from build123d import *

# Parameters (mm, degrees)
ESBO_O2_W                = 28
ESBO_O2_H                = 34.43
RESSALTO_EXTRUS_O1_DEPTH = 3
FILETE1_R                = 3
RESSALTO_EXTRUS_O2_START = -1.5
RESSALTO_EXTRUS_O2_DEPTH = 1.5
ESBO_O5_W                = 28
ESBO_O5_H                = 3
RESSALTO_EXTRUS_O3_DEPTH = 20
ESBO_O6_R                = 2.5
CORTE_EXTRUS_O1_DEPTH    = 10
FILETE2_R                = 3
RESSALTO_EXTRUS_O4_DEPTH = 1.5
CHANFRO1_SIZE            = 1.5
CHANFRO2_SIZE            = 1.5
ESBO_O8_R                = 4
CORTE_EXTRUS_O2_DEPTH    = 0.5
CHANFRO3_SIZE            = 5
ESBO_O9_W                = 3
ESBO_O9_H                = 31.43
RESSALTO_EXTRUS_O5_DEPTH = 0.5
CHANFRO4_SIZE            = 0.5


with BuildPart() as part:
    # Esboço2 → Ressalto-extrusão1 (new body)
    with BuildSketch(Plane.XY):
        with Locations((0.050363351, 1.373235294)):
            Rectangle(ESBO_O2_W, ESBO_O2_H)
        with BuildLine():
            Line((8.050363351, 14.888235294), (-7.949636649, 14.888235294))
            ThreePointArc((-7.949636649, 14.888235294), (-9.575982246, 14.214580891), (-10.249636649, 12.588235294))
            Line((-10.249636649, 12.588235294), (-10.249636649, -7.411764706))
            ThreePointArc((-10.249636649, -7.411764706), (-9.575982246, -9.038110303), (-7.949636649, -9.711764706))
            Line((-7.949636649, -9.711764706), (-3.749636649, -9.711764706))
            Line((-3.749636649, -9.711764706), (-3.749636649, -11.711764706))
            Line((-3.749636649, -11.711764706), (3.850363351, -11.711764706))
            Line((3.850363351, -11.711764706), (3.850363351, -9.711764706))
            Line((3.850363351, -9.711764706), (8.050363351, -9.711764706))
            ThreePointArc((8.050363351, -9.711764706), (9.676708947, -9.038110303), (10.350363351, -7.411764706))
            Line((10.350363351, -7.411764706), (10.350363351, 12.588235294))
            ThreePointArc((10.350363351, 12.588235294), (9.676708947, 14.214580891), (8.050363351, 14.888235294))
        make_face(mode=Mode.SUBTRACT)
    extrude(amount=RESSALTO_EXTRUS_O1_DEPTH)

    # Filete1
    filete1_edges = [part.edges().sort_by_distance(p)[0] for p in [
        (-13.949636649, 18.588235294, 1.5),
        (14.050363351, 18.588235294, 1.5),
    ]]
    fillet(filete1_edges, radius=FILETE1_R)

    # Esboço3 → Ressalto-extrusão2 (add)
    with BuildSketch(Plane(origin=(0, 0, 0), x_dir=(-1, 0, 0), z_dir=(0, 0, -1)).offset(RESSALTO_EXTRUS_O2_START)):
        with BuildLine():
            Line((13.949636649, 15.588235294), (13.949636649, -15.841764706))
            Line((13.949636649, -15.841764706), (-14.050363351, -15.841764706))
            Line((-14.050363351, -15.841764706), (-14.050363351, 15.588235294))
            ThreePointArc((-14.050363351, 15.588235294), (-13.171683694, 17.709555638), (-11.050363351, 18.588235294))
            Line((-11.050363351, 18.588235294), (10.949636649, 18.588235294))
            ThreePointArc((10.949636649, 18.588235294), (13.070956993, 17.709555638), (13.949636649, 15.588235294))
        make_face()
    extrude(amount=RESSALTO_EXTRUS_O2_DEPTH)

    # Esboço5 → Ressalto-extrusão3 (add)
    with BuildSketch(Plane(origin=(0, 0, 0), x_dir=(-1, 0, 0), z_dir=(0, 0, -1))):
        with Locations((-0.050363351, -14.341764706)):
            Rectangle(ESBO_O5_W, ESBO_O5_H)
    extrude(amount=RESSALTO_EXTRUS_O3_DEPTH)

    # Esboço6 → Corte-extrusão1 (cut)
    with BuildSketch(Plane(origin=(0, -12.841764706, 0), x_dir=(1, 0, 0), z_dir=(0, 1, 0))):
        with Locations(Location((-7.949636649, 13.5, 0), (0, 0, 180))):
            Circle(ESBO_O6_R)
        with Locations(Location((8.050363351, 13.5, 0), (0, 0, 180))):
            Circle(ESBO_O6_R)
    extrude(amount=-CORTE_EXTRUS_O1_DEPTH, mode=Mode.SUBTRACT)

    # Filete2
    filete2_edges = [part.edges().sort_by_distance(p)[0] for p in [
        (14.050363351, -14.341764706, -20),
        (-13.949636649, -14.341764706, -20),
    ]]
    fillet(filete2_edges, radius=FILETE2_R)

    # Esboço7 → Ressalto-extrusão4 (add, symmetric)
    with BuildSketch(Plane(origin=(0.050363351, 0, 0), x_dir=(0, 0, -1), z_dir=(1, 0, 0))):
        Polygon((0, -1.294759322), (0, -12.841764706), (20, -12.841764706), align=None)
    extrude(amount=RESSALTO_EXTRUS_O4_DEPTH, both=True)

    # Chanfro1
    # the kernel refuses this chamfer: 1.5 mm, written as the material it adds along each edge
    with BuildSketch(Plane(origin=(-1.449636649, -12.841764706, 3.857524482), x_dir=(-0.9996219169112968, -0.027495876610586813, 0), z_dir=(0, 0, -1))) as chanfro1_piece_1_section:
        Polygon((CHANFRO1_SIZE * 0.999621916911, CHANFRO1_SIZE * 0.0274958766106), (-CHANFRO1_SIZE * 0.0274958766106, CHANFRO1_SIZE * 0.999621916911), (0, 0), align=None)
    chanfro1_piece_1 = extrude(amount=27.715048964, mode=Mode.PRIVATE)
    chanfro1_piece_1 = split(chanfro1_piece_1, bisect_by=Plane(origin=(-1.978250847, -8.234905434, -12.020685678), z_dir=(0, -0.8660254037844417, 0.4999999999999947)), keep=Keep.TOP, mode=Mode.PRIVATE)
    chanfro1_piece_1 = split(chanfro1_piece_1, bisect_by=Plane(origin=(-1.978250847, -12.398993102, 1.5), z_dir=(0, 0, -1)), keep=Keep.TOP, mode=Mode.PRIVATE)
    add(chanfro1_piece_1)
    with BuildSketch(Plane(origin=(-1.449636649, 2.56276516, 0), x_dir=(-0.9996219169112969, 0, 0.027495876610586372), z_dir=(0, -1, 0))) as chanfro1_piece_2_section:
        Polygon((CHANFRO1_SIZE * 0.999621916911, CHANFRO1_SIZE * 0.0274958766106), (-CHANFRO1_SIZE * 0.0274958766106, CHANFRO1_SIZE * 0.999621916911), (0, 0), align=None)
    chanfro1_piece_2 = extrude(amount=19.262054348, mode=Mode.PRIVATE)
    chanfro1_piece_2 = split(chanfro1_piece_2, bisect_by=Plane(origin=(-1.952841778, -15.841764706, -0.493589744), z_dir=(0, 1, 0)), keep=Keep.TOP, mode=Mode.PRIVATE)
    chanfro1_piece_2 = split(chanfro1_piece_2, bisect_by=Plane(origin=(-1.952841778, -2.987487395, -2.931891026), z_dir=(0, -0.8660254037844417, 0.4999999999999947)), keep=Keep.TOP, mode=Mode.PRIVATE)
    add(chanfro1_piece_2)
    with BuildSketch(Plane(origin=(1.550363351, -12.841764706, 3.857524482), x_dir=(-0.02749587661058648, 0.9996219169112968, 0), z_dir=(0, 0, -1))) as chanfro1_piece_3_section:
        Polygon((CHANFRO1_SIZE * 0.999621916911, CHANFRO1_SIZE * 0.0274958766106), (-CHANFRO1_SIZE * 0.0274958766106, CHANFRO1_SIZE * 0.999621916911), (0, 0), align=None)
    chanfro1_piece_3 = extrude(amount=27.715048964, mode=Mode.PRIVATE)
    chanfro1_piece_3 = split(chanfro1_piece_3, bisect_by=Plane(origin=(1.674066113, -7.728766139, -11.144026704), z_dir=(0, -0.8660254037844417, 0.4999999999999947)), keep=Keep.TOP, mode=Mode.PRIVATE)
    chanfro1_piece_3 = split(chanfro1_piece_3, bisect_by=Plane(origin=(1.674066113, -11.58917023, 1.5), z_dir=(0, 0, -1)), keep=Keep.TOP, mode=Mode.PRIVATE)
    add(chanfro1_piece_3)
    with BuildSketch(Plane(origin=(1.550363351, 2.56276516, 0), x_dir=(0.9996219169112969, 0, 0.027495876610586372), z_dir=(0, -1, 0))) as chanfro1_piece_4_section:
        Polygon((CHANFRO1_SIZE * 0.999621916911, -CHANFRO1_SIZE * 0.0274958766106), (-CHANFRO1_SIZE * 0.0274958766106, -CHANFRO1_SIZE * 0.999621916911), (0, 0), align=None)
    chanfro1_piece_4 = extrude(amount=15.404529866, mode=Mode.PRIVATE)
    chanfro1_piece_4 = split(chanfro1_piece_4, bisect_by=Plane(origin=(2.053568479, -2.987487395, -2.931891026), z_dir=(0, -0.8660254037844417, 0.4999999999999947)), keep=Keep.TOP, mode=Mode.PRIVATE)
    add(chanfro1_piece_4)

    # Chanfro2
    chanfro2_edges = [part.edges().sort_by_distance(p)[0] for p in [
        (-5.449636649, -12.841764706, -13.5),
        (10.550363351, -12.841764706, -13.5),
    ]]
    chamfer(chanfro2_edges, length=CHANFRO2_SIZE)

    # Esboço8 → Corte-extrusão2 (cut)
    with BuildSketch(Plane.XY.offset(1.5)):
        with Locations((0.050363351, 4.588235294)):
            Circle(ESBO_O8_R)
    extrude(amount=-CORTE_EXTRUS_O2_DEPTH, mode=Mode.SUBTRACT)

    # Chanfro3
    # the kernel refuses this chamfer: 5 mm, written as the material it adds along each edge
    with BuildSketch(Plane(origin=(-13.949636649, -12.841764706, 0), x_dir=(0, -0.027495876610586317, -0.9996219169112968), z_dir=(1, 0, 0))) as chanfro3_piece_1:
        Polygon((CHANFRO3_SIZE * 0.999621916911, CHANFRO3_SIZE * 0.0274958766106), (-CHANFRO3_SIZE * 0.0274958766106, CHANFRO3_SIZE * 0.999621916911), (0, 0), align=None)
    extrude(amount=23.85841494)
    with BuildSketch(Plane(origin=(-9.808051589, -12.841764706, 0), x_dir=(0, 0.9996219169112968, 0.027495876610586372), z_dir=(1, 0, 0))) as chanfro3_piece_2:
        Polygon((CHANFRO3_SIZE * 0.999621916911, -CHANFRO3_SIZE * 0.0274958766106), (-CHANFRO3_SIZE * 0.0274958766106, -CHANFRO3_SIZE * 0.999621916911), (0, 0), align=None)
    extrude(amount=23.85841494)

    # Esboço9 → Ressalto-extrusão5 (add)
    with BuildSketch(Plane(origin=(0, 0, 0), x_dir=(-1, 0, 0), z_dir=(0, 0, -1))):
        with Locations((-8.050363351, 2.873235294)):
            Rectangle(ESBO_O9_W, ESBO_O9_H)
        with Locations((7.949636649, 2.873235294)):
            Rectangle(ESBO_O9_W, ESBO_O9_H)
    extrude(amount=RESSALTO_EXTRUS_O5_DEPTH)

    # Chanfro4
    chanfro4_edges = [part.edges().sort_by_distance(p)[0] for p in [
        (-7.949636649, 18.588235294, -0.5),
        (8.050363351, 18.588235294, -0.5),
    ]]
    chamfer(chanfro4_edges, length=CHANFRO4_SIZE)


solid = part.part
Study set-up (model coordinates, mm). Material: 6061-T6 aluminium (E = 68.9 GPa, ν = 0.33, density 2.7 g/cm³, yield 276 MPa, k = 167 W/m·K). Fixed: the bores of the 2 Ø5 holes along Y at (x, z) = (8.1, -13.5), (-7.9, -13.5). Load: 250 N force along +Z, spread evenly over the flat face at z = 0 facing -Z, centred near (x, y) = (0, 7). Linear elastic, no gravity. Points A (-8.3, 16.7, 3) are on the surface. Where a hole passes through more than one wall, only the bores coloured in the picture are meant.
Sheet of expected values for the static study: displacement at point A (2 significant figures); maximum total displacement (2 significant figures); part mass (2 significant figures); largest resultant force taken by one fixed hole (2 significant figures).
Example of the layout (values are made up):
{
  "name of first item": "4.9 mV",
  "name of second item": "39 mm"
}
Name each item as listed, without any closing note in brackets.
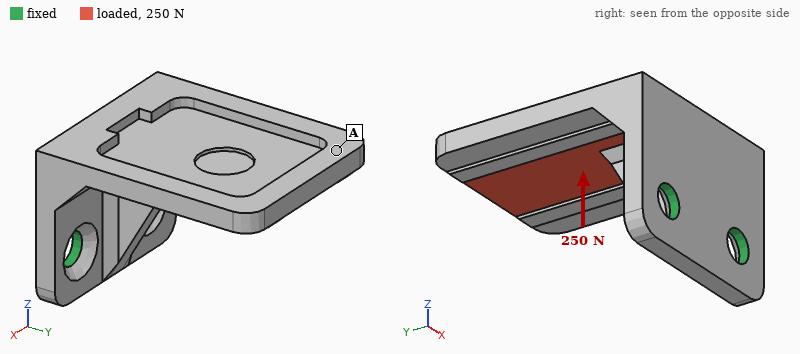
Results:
{
  "displacement at point A": "0.41 mm",
  "maximum total displacement": "0.45 mm",
  "part mass": "12 g",
  "largest resultant force taken by one fixed hole": "130 N"
}
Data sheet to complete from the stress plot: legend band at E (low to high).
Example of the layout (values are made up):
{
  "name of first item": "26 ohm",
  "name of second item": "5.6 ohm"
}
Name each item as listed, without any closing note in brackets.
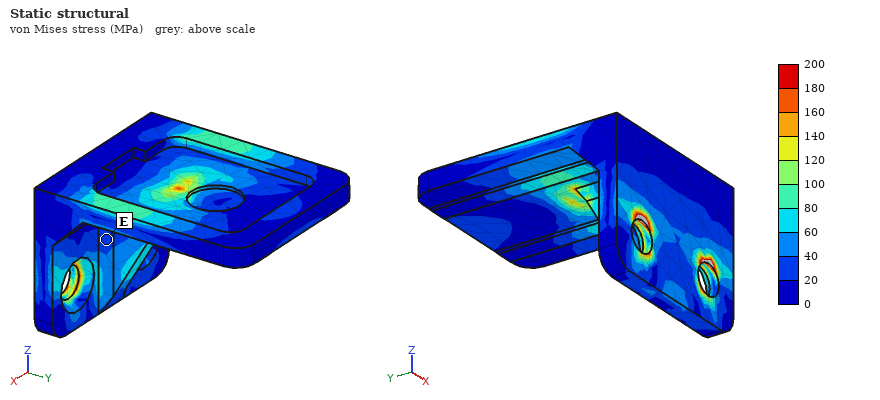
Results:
{
  "legend band at E": "20 to 40 MPa"
}
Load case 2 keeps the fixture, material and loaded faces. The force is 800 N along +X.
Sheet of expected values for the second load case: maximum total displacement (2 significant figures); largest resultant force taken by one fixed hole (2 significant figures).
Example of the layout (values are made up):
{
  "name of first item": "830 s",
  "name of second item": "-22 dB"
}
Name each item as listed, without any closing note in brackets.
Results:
{
  "maximum total displacement": "0.31 mm",
  "largest resultant force taken by one fixed hole": "1.3 kN"
}
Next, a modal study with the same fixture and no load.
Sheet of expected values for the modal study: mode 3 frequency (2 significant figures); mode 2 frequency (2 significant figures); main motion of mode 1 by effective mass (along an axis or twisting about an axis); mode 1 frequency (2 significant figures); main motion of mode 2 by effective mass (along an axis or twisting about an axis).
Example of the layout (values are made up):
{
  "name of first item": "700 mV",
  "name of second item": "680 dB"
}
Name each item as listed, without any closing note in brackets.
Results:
{
  "mode 3 frequency": "5100 Hz",
  "mode 2 frequency": "4300 Hz",
  "main motion of mode 1 by effective mass": "along Z",
  "mode 1 frequency": "2100 Hz",
  "main motion of mode 2 by effective mass": "along X"
}
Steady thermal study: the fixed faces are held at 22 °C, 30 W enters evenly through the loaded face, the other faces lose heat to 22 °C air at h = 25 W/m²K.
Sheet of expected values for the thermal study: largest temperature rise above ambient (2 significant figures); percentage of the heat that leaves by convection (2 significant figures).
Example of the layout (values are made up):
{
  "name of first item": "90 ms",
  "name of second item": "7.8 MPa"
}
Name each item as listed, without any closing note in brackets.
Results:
{
  "largest temperature rise above ambient": "72 K",
  "percentage of the heat that leaves by convection": "8.9 %"
}
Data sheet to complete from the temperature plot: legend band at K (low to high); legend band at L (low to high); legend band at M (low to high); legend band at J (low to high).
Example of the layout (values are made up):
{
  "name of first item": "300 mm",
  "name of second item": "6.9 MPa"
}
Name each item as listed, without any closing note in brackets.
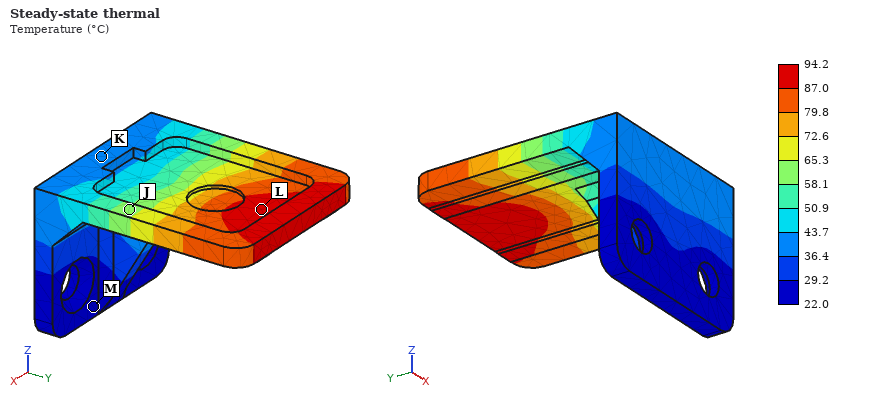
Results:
{
  "legend band at K": "36.4 to 43.7 °C",
  "legend band at L": "87.0 to 94.2 °C",
  "legend band at M": "22.0 to 29.2 °C",
  "legend band at J": "58.1 to 65.3 °C"
}
